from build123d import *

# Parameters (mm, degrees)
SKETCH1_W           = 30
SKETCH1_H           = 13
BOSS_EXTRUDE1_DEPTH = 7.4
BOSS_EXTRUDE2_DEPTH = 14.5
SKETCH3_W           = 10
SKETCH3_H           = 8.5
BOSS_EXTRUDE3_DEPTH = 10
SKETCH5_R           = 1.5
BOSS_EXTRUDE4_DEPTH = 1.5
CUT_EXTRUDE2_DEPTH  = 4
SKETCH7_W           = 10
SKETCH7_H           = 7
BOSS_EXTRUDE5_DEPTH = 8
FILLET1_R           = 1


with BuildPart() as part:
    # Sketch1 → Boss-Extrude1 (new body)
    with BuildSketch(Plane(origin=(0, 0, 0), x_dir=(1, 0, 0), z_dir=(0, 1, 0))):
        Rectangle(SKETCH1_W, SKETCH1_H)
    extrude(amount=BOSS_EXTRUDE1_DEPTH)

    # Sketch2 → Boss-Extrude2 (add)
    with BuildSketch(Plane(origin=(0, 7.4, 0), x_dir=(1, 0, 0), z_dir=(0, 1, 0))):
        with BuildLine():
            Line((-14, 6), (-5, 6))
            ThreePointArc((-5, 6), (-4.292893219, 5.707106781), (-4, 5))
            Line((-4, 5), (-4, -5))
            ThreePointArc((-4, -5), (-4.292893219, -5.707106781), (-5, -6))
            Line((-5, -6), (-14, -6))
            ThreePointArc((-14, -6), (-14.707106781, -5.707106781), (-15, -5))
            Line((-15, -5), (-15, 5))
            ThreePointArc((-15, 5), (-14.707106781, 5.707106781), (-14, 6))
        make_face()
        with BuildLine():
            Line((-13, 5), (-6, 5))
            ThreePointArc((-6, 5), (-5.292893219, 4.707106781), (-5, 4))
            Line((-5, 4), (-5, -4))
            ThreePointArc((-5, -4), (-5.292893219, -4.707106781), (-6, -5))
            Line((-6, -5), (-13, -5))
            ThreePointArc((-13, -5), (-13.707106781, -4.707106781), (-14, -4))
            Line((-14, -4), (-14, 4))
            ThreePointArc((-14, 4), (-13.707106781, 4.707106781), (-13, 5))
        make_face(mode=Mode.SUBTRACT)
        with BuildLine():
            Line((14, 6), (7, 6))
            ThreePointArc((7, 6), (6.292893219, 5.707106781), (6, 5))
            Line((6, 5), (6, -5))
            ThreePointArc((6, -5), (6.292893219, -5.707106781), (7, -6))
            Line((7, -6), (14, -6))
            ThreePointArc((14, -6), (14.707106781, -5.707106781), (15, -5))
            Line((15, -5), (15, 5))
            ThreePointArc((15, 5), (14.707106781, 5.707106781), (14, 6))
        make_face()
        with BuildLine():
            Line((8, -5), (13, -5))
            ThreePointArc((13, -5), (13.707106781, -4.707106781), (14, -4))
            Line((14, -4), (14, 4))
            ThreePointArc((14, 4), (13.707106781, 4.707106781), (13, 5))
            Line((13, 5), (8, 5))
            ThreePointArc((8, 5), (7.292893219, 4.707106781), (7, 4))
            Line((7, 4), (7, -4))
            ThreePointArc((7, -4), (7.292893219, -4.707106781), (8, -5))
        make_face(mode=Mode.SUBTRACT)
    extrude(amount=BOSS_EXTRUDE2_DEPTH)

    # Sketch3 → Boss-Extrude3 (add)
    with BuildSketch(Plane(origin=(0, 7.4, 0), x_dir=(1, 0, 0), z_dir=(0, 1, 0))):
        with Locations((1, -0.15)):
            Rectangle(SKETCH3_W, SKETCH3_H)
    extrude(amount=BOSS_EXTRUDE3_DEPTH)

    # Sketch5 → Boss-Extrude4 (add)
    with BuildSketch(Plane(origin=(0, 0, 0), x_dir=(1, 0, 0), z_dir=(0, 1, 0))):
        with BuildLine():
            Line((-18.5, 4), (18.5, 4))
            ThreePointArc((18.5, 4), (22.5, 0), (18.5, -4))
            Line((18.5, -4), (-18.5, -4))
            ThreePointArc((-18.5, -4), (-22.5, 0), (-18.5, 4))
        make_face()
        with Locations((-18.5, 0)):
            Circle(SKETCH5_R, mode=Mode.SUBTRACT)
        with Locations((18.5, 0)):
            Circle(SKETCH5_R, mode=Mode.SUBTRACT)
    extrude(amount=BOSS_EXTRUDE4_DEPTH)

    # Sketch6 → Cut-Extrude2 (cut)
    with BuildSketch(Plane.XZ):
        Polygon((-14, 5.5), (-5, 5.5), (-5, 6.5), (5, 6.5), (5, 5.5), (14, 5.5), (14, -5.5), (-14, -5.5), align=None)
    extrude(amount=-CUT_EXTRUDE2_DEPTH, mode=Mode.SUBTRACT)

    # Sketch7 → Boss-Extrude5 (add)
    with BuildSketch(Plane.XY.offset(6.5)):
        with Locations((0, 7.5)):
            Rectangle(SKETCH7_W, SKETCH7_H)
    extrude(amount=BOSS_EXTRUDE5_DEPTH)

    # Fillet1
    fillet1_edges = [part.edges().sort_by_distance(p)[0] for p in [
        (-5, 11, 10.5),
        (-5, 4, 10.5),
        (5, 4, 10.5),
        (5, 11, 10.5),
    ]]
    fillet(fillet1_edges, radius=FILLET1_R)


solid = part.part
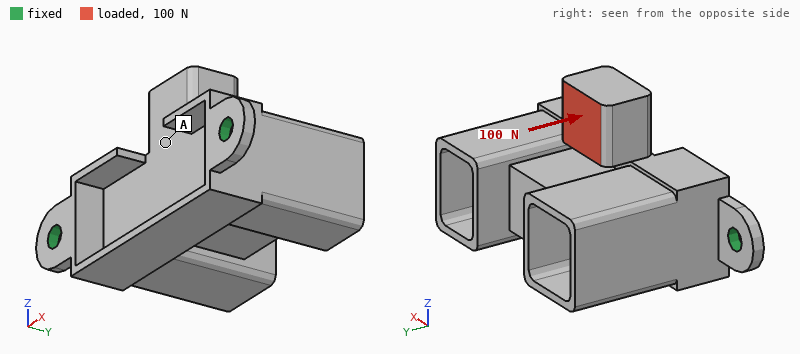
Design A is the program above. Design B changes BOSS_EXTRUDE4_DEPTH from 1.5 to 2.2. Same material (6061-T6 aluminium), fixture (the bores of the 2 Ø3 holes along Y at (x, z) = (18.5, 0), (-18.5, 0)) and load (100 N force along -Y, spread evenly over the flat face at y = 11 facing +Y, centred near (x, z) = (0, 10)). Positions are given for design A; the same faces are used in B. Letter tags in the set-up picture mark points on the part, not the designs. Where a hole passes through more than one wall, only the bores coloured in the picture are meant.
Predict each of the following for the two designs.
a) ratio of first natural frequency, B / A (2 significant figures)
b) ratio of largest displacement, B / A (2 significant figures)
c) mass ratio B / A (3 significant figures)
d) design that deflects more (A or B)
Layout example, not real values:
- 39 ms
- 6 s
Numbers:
- 1.5
- 0.51
- 1.01
- A
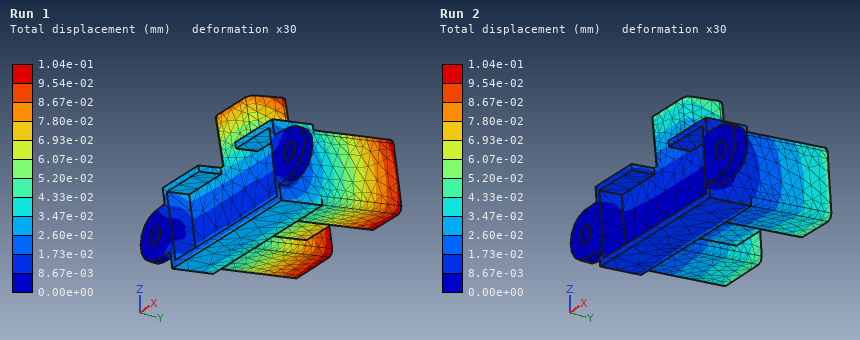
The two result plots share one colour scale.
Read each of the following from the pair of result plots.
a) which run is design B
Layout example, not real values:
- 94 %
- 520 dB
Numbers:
- Run 2
